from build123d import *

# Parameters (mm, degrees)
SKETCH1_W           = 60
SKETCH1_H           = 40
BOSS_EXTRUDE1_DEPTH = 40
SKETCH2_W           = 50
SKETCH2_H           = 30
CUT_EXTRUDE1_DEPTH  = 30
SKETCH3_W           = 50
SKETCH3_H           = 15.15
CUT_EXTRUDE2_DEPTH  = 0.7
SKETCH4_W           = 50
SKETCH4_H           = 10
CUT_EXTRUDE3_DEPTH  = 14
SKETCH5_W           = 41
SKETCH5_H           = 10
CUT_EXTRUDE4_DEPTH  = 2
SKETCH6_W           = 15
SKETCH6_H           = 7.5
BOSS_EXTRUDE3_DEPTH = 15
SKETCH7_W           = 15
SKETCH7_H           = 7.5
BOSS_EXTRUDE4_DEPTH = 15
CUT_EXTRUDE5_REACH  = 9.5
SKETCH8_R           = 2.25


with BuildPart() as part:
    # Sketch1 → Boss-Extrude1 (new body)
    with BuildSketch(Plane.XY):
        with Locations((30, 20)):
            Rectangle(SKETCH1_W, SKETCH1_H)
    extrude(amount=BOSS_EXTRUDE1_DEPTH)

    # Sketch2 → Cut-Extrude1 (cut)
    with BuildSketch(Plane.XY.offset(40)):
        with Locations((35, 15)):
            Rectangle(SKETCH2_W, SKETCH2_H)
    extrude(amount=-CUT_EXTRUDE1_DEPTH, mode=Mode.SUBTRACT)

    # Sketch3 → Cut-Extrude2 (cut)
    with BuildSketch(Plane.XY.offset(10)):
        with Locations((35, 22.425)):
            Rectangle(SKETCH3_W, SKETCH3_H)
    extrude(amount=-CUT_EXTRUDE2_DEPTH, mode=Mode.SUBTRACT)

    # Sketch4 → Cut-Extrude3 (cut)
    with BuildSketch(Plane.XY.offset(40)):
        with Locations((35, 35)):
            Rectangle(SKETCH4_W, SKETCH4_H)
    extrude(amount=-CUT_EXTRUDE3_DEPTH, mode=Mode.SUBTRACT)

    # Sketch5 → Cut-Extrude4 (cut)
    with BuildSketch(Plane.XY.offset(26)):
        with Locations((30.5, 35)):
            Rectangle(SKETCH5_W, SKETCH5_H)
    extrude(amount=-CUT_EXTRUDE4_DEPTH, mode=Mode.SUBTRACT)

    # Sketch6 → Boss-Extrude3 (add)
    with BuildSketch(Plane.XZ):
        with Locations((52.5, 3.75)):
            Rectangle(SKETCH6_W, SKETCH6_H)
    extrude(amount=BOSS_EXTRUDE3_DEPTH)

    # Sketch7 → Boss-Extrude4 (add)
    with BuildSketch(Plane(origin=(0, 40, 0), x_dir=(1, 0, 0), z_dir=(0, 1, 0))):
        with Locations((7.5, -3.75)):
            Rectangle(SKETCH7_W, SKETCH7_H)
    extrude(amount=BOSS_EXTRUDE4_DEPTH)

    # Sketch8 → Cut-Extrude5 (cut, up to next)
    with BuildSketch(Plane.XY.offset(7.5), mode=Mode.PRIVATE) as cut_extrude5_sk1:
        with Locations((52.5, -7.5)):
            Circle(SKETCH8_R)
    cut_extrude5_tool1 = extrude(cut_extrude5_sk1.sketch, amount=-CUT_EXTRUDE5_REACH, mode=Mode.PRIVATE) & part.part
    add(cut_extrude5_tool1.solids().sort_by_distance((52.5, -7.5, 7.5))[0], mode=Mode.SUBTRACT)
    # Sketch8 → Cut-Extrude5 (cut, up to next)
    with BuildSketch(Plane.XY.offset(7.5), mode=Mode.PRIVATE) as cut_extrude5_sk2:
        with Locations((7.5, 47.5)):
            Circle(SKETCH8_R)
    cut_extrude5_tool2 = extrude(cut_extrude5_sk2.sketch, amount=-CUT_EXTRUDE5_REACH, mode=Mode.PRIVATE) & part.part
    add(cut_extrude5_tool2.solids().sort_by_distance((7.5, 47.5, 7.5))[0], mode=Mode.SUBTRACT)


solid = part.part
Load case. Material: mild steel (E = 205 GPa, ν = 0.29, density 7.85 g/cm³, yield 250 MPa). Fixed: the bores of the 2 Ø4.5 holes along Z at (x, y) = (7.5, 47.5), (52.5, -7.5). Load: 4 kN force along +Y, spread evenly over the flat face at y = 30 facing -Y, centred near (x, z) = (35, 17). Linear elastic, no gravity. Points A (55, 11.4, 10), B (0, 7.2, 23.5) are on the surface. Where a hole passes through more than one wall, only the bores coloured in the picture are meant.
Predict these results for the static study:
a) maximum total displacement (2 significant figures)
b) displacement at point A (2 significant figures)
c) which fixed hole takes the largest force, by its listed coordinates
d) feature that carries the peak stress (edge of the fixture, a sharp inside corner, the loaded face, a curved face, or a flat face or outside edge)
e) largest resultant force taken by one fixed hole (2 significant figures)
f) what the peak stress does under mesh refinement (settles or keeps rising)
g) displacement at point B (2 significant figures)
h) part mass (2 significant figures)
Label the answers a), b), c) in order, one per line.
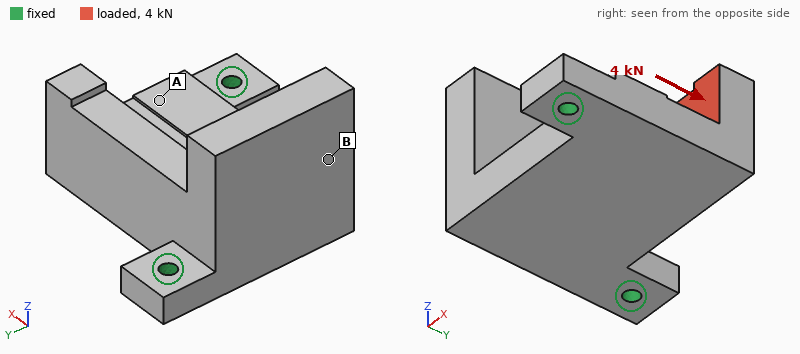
a) 99 µm
b) 17 µm
c) (52.5, -7.5)
d) edge of the fixture
e) 2.4 kN
f) keeps rising
g) 71 µm
h) 360 g
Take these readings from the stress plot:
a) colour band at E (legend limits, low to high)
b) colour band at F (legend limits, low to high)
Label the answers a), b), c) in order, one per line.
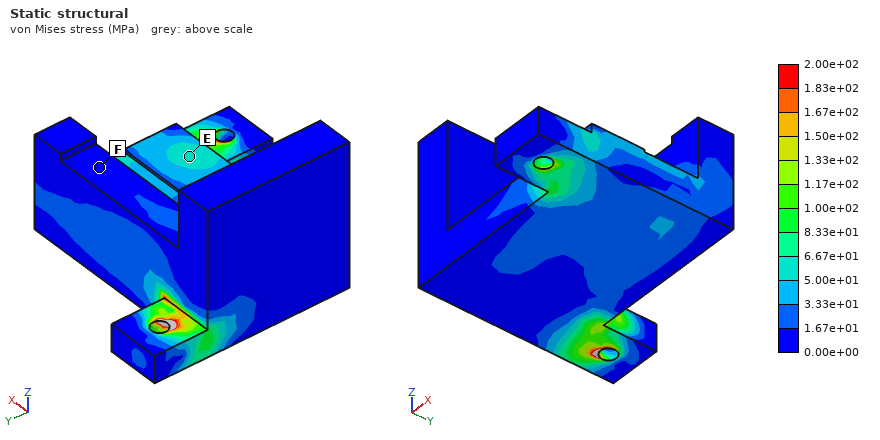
a) 5.00e+01 to 6.67e+01 MPa
b) 0.00e+00 to 1.67e+01 MPa
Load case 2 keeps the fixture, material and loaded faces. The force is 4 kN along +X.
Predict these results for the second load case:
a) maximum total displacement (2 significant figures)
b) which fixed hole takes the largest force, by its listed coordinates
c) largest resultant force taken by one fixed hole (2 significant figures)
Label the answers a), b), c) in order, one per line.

a) 88 µm
b) (7.5, 47.5)
c) 2.5 kN
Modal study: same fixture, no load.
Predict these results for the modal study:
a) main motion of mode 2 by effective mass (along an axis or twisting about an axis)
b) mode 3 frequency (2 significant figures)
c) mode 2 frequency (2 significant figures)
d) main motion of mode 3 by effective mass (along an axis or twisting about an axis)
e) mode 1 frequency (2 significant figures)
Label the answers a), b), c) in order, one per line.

a) along Z
b) 6200 Hz
c) 3600 Hz
d) along X
e) 1800 Hz
